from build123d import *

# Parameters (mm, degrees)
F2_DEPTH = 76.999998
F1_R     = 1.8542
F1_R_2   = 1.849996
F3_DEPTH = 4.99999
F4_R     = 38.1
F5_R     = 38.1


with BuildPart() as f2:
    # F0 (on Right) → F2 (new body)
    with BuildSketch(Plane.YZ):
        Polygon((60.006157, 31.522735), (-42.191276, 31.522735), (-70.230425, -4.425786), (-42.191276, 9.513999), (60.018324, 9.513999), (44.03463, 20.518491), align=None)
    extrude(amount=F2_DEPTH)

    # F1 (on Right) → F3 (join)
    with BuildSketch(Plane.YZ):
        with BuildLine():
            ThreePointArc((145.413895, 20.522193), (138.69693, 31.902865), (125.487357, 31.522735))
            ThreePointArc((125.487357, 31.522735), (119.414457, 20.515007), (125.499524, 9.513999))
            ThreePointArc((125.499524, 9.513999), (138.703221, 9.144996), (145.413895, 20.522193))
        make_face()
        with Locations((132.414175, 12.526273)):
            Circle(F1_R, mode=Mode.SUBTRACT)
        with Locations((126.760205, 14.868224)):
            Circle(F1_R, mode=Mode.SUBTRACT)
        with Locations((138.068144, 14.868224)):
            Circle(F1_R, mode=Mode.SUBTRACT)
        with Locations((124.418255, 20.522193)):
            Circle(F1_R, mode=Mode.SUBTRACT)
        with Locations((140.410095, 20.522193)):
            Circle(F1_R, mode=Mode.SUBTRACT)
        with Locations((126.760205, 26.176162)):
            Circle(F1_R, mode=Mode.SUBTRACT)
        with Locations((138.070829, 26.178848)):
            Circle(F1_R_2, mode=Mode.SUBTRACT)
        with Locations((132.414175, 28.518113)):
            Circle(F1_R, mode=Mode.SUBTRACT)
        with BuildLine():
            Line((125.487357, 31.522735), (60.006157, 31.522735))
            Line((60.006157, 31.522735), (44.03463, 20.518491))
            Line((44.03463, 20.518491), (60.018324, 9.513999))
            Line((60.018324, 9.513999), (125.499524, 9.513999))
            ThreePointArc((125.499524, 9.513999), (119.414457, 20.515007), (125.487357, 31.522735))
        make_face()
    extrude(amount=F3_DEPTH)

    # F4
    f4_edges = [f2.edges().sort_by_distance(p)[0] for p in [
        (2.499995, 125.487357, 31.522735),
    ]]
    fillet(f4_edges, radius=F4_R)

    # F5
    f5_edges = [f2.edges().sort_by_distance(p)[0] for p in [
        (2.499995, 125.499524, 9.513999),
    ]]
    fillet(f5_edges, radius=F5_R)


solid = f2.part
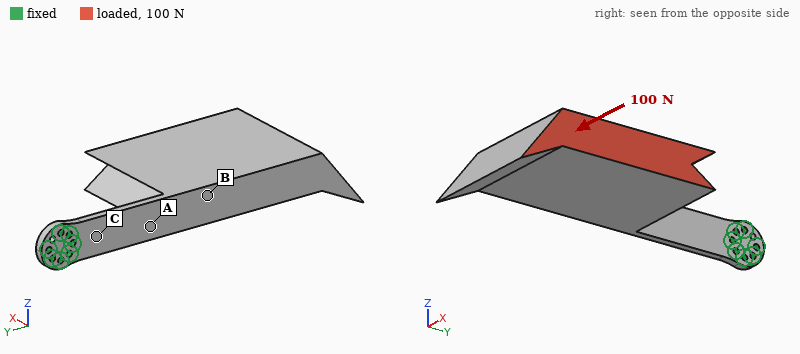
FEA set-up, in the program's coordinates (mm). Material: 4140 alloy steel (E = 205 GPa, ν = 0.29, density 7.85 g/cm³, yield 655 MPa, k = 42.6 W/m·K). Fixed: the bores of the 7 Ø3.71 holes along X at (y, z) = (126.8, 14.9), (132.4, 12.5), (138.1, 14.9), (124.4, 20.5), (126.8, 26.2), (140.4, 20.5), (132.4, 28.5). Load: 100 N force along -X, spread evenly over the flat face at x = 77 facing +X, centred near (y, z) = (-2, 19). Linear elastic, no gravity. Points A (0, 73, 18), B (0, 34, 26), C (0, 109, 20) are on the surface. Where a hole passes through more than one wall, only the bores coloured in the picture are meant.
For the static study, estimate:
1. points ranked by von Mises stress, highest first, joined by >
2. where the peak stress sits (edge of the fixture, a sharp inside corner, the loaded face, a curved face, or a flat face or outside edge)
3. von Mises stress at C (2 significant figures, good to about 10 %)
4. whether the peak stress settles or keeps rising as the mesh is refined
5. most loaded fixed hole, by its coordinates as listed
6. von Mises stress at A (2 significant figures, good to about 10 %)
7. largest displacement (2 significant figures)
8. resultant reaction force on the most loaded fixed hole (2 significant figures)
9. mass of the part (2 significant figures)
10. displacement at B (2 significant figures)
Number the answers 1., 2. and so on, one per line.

1. C > A > B
2. edge of the fixture
3. 120 MPa
4. keeps rising
5. (124.4, 20.5)
6. 82 MPa
7. 2.5 mm
8. 650 N
9. 1.5 kg
10. 0.80 mm
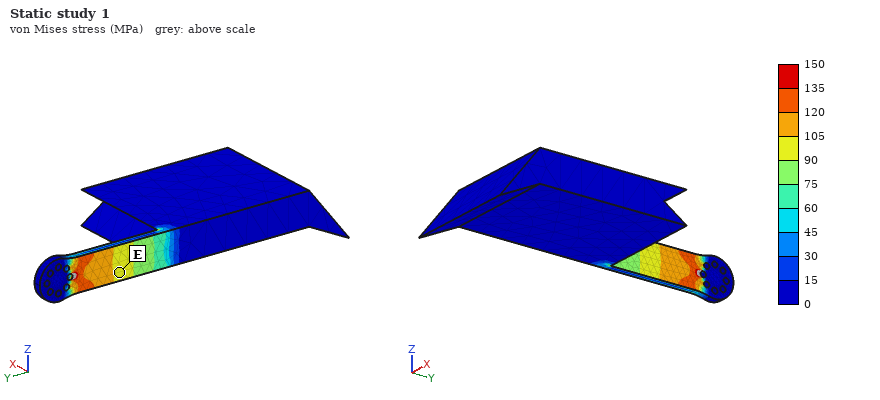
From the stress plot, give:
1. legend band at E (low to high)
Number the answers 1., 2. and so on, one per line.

1. 90 to 105 MPa
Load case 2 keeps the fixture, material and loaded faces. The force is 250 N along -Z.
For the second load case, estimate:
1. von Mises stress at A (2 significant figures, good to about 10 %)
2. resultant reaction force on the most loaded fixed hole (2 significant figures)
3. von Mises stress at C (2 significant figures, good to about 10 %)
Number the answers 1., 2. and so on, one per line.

1. 190 MPa
2. 1.8 kN
3. 190 MPa
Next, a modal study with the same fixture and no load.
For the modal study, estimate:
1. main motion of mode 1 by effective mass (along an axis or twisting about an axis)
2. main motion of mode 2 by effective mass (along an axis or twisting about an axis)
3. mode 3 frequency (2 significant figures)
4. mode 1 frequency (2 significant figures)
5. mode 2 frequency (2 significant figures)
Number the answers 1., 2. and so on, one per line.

1. along X
2. along Z
3. 270 Hz
4. 32 Hz
5. 85 Hz
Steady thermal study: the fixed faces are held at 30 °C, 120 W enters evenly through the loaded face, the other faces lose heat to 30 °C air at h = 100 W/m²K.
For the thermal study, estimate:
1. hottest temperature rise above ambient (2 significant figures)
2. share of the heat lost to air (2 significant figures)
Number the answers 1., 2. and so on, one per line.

1. 78 K
2. 99 %
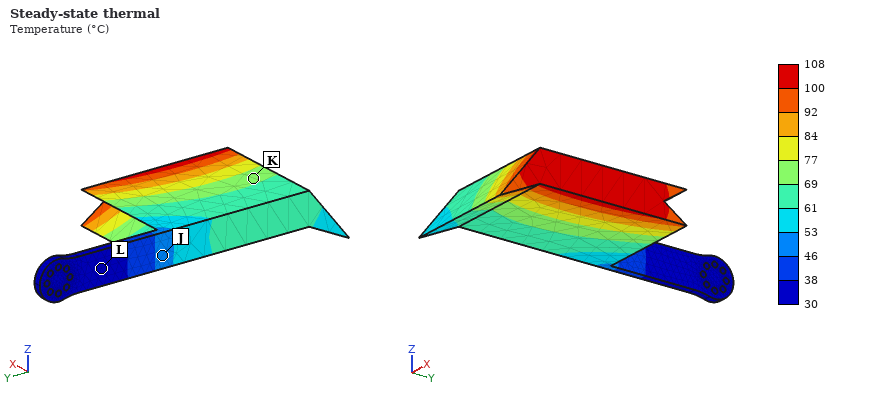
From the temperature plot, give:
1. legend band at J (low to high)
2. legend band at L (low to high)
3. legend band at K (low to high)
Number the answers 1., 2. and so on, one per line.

1. 46 to 53 °C
2. 30 to 38 °C
3. 69 to 77 °C
